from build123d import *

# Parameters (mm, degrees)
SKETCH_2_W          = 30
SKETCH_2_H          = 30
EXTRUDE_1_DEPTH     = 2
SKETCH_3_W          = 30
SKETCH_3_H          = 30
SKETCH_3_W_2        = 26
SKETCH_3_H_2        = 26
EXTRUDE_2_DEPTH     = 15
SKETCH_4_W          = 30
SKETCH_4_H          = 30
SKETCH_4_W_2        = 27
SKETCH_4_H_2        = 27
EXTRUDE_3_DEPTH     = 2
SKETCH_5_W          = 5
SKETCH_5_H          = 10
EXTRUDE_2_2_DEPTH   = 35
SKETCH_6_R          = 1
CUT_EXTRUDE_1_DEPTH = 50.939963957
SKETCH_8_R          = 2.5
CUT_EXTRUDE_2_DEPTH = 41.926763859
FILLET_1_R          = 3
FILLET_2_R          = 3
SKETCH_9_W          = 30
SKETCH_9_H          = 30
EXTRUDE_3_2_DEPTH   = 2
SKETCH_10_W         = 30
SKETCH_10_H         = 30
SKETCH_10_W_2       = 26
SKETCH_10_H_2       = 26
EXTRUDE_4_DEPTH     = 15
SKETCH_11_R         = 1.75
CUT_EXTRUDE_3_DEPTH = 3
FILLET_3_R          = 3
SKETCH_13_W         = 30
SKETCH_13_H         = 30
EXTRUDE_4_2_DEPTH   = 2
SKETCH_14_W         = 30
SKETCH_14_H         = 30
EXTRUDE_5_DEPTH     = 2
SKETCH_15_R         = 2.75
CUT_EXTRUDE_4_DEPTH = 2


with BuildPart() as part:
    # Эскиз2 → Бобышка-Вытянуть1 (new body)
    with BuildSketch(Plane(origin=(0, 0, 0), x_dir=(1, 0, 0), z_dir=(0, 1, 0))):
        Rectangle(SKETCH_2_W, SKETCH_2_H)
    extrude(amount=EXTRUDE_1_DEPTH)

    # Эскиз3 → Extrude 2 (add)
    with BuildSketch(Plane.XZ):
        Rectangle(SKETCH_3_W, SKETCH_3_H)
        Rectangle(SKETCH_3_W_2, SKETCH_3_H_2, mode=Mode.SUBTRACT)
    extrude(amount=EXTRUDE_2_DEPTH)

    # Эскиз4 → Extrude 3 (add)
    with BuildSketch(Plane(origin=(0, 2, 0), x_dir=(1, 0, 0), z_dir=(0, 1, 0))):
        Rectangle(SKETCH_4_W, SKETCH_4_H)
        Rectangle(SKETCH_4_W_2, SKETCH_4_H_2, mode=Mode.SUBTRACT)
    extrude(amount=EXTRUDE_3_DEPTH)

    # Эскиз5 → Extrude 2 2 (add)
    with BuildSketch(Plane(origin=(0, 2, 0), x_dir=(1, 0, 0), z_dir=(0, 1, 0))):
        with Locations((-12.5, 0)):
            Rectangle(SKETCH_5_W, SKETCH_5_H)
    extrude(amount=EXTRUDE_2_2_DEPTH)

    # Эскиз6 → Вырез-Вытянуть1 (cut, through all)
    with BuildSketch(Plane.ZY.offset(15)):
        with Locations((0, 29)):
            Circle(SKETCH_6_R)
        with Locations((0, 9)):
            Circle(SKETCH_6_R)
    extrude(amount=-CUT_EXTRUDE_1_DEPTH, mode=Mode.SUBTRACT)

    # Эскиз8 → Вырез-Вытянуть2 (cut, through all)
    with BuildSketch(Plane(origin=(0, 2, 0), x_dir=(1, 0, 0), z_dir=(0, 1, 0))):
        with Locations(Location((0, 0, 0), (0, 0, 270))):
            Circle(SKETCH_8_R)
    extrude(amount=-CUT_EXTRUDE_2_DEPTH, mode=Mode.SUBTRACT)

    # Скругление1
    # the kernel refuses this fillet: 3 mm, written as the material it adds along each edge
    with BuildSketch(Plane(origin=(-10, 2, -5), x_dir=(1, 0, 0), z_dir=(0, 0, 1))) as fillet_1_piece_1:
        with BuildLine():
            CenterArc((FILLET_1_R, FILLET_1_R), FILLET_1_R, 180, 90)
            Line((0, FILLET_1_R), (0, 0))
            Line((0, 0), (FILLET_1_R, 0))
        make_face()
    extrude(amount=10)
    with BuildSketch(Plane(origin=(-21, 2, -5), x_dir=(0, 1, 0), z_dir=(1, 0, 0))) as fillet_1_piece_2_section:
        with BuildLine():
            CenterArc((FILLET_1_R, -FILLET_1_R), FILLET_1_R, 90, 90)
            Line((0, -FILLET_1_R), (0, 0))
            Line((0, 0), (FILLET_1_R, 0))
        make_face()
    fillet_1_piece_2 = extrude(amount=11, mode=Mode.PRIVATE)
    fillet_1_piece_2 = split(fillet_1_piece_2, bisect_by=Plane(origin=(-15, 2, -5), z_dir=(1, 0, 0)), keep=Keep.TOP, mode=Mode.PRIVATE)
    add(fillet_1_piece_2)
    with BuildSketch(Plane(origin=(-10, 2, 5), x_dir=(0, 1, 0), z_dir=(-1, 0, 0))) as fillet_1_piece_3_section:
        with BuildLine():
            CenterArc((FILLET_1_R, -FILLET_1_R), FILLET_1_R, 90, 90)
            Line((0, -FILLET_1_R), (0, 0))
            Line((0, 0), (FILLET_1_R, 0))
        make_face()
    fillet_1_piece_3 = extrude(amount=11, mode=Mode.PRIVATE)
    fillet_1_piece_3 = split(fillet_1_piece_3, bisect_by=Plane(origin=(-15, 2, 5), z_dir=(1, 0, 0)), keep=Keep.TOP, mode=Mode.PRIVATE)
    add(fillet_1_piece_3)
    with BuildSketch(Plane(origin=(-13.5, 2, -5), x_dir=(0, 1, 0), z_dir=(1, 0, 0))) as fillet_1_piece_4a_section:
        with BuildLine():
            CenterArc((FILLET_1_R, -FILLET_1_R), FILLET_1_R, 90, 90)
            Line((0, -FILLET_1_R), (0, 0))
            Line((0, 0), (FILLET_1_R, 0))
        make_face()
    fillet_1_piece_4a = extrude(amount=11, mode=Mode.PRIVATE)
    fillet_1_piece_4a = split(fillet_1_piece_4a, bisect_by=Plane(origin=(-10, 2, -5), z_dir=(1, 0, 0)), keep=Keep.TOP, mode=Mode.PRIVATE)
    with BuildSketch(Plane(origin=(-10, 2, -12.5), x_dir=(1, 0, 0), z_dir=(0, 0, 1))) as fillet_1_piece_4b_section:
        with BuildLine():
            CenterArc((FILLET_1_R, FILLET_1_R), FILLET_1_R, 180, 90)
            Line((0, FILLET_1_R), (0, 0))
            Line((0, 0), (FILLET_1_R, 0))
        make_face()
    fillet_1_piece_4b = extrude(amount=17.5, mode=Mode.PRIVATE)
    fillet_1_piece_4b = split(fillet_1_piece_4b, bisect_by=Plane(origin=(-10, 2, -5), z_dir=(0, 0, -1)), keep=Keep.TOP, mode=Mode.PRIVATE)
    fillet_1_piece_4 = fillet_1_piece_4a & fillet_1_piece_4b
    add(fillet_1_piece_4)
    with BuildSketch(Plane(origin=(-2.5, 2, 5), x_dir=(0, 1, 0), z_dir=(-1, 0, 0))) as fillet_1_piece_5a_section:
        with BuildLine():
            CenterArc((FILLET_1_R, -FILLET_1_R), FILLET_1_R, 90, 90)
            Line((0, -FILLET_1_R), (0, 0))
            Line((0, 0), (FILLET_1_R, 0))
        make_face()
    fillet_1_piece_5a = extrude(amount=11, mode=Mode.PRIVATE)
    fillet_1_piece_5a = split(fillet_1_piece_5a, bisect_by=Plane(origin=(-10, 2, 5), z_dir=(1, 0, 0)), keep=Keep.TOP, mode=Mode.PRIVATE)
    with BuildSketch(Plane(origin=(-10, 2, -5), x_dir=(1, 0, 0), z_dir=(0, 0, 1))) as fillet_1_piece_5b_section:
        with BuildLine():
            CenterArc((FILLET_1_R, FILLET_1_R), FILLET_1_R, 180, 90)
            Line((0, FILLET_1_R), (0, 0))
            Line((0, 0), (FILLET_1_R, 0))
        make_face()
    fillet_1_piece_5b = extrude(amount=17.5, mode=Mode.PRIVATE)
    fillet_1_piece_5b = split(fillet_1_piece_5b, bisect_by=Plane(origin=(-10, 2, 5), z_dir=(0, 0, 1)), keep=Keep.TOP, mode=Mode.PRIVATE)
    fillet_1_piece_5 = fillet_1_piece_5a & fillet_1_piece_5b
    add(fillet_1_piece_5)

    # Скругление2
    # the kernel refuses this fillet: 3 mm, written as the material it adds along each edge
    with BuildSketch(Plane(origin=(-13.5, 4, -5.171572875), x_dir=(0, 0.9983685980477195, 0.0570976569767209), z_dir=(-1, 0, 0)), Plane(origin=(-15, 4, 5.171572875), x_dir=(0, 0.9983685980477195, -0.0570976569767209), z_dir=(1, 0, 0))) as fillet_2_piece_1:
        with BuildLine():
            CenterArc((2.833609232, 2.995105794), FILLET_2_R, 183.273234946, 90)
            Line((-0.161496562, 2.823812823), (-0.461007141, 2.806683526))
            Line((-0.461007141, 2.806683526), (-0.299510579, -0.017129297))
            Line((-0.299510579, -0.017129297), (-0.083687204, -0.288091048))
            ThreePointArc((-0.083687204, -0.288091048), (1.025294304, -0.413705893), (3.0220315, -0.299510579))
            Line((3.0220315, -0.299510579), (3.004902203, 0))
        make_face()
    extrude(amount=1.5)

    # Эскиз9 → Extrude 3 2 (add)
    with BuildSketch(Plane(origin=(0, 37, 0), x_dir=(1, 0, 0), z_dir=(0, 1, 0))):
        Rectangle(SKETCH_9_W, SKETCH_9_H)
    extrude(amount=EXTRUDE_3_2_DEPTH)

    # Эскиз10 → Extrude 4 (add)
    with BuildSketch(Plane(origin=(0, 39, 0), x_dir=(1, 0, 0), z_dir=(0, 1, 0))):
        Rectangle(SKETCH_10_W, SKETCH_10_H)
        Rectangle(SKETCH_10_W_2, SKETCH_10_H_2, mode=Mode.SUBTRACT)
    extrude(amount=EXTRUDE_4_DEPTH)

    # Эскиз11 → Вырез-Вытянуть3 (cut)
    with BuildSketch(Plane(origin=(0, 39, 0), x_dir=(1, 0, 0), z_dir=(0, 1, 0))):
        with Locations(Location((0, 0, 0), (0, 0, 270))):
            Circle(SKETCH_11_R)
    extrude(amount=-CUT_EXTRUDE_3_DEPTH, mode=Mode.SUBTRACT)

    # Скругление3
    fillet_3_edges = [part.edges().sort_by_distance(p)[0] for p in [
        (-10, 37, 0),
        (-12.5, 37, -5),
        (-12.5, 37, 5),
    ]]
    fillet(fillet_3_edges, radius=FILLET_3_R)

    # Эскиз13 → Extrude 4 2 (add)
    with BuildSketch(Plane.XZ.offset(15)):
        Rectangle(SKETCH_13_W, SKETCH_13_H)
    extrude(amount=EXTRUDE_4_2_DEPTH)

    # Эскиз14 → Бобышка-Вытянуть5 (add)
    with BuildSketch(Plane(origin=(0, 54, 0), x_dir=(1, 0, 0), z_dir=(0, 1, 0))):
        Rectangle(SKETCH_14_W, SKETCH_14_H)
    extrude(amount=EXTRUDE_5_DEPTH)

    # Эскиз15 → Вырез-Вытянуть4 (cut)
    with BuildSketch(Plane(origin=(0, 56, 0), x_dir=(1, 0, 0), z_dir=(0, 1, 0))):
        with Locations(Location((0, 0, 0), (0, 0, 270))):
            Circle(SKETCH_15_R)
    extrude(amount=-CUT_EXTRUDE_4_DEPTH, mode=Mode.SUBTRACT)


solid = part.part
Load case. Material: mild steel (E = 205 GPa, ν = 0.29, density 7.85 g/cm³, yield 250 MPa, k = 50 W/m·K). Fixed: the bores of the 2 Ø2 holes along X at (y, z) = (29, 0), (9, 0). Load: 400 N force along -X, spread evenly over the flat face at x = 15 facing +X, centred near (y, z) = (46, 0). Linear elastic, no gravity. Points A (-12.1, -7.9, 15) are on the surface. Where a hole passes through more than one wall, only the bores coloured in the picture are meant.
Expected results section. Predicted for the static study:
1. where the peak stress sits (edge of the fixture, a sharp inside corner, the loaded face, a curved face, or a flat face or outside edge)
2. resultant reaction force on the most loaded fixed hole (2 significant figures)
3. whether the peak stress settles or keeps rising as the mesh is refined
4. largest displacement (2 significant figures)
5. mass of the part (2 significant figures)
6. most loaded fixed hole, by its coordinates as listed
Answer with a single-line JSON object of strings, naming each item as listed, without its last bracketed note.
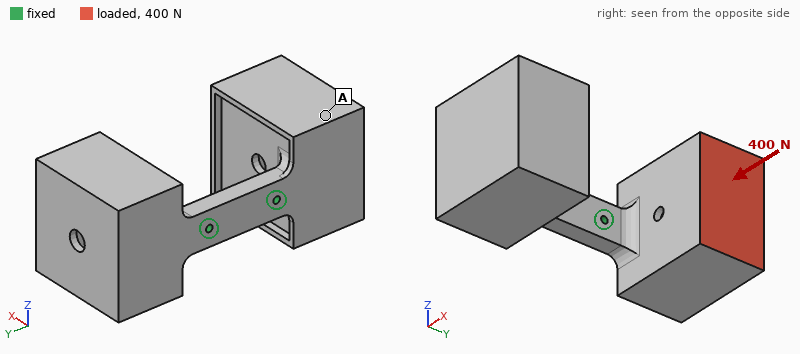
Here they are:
{"where the peak stress sits": "edge of the fixture", "resultant reaction force on the most loaded fixed hole": "480 N", "whether the peak stress settles or keeps rising as the mesh is refined": "keeps rising", "largest displacement": "0.12 mm", "mass of the part": "130 g", "most loaded fixed hole, by its coordinates as listed": "(29, 0)"}
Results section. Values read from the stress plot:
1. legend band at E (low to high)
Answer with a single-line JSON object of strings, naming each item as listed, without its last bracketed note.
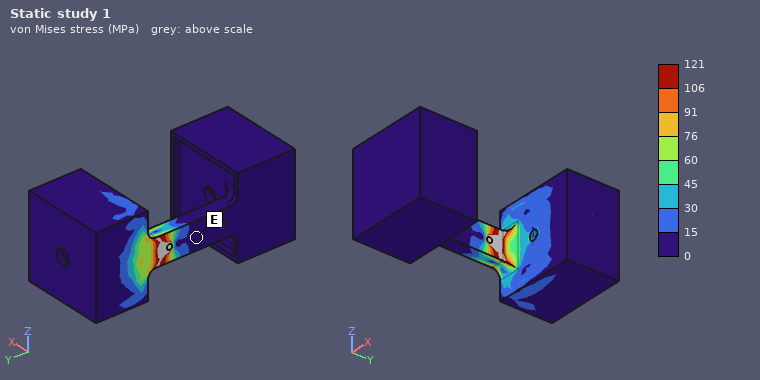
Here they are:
{"legend band at E": "0 to 15 MPa"}
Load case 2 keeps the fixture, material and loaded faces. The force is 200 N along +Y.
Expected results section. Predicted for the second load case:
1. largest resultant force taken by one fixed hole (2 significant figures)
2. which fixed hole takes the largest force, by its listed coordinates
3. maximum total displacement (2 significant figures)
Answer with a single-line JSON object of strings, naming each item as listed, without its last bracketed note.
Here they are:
{"largest resultant force taken by one fixed hole": "190 N", "which fixed hole takes the largest force, by its listed coordinates": "(29, 0)", "maximum total displacement": "0.15 mm"}
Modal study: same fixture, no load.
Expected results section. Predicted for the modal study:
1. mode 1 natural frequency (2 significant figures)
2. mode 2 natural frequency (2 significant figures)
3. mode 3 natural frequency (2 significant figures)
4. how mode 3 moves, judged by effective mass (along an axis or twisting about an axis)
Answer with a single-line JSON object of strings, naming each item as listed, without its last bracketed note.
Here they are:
{"mode 1 natural frequency": "1200 Hz", "mode 2 natural frequency": "1200 Hz", "mode 3 natural frequency": "1700 Hz", "how mode 3 moves, judged by effective mass": "along Z"}
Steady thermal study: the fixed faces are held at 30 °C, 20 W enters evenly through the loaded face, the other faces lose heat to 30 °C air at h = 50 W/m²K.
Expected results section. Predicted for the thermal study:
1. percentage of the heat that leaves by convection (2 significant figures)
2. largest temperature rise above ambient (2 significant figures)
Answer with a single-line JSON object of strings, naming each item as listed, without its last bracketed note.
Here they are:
{"percentage of the heat that leaves by convection": "71 %", "largest temperature rise above ambient": "76 K"}
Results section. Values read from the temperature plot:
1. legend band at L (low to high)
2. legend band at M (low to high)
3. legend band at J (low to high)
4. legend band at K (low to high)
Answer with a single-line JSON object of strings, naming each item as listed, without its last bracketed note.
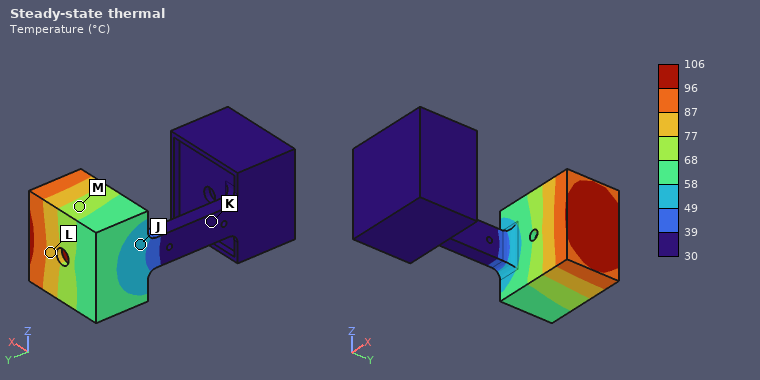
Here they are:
{"legend band at L": "77 to 87 °C", "legend band at M": "68 to 77 °C", "legend band at J": "49 to 58 °C", "legend band at K": "30 to 39 °C"}
